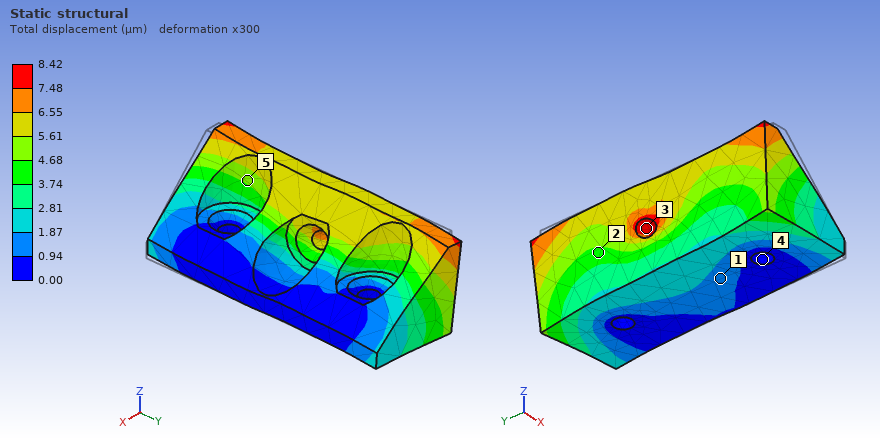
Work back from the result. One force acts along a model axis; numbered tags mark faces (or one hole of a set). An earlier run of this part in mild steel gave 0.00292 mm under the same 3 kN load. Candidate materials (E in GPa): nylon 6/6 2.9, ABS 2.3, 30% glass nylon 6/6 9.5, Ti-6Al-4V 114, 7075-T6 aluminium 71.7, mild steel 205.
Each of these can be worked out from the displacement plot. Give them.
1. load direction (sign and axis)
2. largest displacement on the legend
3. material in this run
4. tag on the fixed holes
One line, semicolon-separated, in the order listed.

+Y; 8.42 µm; 7075-T6 aluminium; 4
